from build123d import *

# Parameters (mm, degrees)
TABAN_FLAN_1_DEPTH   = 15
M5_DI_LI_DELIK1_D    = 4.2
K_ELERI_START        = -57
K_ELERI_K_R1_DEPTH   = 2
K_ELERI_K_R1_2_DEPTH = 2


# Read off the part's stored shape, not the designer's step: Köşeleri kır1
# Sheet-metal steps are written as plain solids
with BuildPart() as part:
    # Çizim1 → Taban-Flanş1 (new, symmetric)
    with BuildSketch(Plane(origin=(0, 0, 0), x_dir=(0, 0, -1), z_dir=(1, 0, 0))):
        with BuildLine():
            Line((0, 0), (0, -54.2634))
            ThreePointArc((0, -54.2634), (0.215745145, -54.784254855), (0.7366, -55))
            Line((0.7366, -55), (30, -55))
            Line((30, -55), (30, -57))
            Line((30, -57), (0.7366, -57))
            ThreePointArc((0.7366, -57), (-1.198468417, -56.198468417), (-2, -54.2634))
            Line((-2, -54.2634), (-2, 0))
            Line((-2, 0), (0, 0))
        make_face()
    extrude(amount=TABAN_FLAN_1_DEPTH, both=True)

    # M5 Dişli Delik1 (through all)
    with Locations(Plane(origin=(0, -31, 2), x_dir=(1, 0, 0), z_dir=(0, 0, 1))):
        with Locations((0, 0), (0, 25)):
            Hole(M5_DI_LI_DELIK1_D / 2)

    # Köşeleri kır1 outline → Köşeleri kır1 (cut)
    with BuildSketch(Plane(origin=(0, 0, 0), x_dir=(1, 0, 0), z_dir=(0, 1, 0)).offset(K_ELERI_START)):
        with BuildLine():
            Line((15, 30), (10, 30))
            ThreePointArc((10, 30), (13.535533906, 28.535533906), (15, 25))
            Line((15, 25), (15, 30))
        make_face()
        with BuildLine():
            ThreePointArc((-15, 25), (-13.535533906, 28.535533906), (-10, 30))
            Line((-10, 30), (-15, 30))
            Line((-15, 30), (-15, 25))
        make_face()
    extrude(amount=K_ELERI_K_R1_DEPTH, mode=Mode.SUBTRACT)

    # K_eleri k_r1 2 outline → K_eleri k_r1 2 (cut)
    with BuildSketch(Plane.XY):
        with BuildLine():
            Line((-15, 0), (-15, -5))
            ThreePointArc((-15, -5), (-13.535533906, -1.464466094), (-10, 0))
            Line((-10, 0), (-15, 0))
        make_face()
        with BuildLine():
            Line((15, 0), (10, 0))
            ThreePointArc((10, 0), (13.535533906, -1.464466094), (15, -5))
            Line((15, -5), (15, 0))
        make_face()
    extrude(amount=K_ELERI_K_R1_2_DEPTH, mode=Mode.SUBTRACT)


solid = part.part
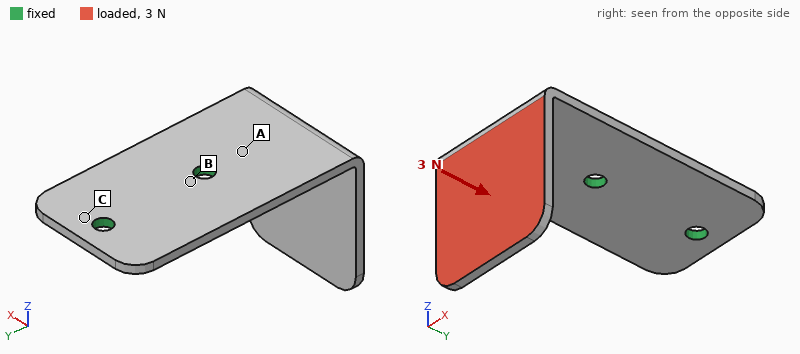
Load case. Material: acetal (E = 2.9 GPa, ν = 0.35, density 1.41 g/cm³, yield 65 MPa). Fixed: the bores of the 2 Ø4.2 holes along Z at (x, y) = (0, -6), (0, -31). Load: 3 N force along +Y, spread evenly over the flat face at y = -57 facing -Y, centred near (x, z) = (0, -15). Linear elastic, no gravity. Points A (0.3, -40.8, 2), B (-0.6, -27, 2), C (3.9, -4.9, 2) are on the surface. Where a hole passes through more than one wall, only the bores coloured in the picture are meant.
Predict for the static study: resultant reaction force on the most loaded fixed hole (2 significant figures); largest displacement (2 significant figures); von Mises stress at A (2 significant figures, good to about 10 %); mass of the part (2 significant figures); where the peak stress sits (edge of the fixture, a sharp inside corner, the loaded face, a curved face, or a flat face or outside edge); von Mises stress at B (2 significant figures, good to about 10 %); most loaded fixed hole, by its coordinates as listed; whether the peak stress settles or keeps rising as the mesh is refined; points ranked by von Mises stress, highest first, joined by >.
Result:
2.5 N
0.83 mm
2.1 MPa
7.2 g
edge of the fixture
0.65 MPa
(0, -31)
keeps rising
A > B > C
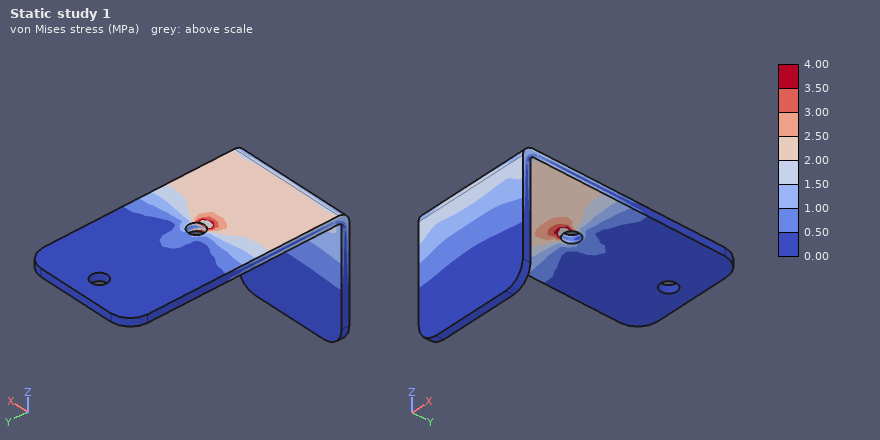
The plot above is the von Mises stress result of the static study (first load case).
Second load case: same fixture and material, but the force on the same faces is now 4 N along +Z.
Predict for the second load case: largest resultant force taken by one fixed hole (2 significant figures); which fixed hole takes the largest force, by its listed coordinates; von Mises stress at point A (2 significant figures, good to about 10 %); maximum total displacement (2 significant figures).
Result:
5.0 N
(0, -31)
3.0 MPa
0.81 mm
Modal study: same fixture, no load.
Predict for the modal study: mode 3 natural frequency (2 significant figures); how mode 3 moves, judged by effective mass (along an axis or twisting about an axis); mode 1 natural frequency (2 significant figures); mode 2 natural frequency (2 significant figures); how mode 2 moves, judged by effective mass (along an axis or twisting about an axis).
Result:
560 Hz
along Z
200 Hz
310 Hz
along X
